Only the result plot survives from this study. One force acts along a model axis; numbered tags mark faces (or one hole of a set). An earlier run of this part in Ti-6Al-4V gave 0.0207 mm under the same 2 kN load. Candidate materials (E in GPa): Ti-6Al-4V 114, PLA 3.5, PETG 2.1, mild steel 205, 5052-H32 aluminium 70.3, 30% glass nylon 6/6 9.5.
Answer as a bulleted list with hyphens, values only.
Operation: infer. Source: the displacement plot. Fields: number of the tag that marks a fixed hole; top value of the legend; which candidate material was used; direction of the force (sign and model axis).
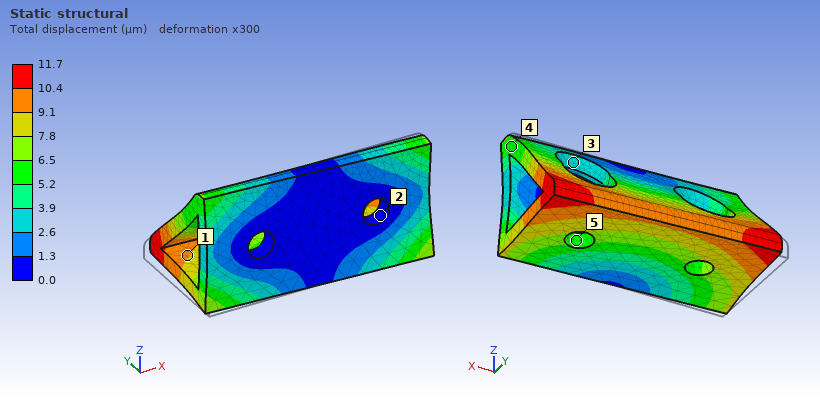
- 2
- 11.7 µm
- mild steel
- +X
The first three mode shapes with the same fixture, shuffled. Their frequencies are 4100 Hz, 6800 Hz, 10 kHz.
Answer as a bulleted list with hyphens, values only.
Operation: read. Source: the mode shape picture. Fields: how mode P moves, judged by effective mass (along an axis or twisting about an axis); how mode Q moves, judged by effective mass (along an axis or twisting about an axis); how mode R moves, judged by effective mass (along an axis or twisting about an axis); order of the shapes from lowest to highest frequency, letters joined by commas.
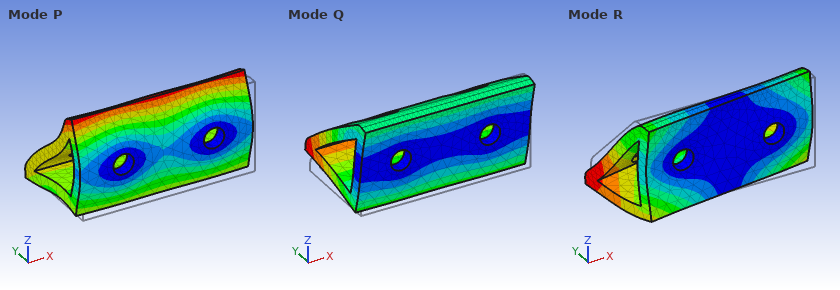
- along Y
- along Z
- along X
- Q, R, P
